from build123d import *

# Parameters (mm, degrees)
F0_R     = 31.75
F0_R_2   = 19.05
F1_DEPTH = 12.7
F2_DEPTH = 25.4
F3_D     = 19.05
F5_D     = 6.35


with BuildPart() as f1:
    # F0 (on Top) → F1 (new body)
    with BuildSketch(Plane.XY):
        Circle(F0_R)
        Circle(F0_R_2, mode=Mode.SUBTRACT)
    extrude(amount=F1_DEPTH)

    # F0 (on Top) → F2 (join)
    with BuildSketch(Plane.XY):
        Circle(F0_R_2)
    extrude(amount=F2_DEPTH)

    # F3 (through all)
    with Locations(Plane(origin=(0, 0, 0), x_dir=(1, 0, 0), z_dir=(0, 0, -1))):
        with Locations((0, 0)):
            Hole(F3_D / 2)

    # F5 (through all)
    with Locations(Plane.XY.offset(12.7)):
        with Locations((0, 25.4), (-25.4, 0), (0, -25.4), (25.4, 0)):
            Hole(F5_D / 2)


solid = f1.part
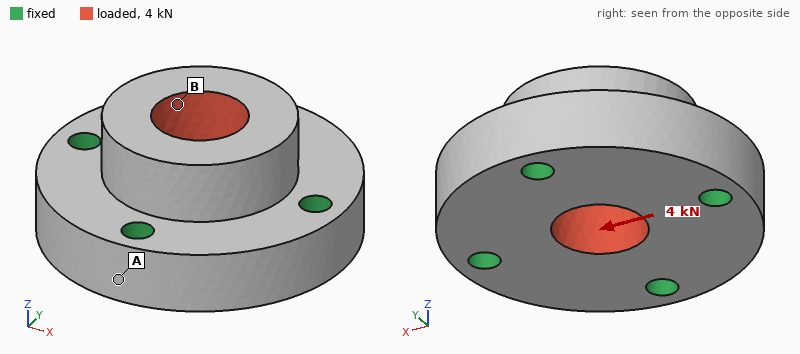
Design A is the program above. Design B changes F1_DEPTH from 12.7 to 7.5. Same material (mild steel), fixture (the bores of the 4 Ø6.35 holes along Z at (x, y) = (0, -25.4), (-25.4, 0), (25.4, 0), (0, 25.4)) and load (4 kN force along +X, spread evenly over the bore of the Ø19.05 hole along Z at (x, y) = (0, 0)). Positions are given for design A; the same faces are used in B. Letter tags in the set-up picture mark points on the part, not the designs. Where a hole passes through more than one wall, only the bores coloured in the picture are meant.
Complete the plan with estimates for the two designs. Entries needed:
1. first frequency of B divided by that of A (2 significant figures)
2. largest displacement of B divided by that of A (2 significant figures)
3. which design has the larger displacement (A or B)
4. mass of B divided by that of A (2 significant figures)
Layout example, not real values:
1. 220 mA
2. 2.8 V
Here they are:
1. 0.68
2. 2.1
3. B
4. 0.78
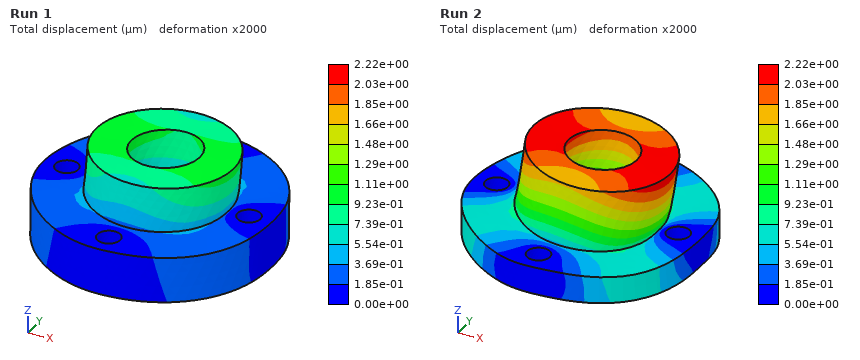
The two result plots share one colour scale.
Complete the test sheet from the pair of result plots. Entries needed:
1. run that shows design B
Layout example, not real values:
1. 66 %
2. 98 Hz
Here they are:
1. Run 2
